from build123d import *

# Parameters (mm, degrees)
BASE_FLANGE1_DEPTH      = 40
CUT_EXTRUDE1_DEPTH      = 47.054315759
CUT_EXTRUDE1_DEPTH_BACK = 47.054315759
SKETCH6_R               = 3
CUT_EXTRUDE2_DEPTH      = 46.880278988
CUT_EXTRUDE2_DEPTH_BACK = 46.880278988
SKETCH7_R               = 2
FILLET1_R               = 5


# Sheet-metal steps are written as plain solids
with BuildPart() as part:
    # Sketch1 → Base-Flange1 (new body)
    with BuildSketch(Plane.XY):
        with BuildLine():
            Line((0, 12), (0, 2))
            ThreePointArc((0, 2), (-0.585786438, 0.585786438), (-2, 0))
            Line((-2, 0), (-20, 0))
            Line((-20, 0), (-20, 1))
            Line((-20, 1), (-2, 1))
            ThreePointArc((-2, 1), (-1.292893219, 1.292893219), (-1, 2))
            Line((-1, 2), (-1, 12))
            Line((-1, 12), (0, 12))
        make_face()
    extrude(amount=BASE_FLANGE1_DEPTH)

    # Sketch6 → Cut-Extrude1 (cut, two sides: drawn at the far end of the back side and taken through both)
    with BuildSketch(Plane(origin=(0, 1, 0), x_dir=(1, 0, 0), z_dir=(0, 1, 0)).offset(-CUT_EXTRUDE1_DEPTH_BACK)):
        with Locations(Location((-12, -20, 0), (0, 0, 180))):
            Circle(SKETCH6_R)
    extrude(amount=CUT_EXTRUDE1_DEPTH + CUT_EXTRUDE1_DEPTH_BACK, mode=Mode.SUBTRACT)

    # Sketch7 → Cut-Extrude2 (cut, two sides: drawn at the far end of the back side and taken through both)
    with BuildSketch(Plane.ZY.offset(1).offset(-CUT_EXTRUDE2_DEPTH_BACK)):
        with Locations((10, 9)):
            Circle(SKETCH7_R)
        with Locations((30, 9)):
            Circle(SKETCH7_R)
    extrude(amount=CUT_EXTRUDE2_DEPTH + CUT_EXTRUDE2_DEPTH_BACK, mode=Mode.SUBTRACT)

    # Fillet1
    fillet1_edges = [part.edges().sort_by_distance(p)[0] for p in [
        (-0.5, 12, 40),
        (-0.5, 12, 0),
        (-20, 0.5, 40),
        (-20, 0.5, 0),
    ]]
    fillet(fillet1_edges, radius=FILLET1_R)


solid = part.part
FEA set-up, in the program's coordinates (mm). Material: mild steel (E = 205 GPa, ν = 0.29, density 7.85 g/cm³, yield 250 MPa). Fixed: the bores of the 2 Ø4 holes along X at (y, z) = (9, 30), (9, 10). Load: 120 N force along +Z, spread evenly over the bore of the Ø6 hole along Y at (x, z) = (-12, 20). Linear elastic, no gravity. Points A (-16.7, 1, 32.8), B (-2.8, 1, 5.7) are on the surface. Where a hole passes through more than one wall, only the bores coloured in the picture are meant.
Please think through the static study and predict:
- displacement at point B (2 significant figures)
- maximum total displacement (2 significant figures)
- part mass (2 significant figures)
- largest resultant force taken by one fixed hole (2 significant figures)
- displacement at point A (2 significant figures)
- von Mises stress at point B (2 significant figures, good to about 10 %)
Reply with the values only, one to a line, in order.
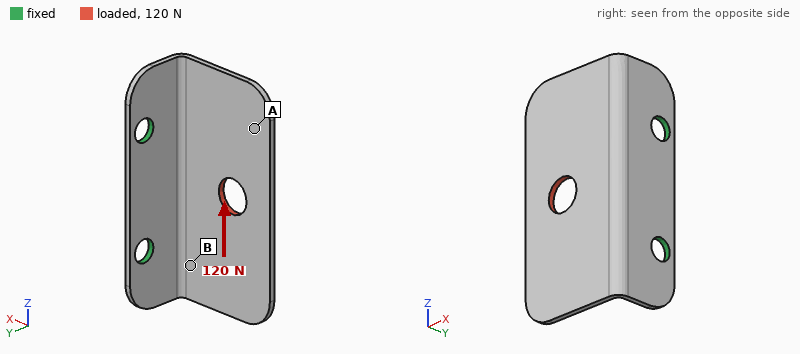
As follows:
25 µm
62 µm
8.9 g
94 N
48 µm
37 MPa
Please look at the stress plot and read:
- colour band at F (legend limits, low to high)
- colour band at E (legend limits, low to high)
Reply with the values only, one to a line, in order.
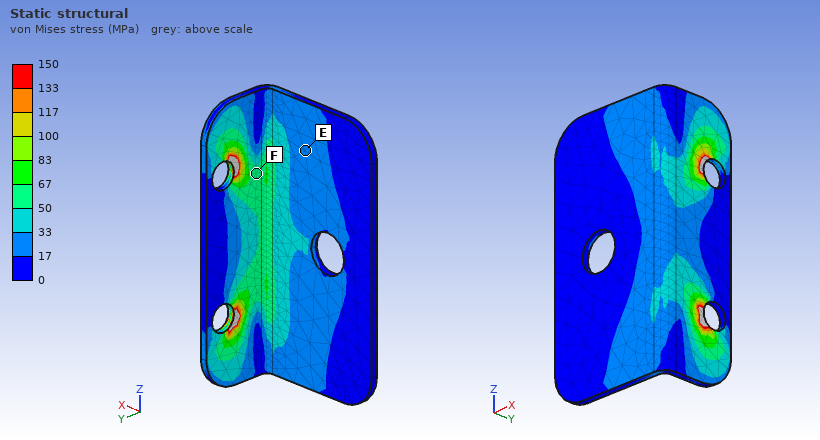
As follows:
50 to 67 MPa
17 to 33 MPa
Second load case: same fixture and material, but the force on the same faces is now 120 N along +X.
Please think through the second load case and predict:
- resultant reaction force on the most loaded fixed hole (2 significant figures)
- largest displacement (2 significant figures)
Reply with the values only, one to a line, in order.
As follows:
60 N
0.11 mm
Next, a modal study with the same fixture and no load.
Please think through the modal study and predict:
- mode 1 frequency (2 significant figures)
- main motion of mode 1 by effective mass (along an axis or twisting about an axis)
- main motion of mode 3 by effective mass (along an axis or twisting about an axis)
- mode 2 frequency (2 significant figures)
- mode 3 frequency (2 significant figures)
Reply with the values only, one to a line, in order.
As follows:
1400 Hz
along Y
along Z
2500 Hz
4300 Hz
